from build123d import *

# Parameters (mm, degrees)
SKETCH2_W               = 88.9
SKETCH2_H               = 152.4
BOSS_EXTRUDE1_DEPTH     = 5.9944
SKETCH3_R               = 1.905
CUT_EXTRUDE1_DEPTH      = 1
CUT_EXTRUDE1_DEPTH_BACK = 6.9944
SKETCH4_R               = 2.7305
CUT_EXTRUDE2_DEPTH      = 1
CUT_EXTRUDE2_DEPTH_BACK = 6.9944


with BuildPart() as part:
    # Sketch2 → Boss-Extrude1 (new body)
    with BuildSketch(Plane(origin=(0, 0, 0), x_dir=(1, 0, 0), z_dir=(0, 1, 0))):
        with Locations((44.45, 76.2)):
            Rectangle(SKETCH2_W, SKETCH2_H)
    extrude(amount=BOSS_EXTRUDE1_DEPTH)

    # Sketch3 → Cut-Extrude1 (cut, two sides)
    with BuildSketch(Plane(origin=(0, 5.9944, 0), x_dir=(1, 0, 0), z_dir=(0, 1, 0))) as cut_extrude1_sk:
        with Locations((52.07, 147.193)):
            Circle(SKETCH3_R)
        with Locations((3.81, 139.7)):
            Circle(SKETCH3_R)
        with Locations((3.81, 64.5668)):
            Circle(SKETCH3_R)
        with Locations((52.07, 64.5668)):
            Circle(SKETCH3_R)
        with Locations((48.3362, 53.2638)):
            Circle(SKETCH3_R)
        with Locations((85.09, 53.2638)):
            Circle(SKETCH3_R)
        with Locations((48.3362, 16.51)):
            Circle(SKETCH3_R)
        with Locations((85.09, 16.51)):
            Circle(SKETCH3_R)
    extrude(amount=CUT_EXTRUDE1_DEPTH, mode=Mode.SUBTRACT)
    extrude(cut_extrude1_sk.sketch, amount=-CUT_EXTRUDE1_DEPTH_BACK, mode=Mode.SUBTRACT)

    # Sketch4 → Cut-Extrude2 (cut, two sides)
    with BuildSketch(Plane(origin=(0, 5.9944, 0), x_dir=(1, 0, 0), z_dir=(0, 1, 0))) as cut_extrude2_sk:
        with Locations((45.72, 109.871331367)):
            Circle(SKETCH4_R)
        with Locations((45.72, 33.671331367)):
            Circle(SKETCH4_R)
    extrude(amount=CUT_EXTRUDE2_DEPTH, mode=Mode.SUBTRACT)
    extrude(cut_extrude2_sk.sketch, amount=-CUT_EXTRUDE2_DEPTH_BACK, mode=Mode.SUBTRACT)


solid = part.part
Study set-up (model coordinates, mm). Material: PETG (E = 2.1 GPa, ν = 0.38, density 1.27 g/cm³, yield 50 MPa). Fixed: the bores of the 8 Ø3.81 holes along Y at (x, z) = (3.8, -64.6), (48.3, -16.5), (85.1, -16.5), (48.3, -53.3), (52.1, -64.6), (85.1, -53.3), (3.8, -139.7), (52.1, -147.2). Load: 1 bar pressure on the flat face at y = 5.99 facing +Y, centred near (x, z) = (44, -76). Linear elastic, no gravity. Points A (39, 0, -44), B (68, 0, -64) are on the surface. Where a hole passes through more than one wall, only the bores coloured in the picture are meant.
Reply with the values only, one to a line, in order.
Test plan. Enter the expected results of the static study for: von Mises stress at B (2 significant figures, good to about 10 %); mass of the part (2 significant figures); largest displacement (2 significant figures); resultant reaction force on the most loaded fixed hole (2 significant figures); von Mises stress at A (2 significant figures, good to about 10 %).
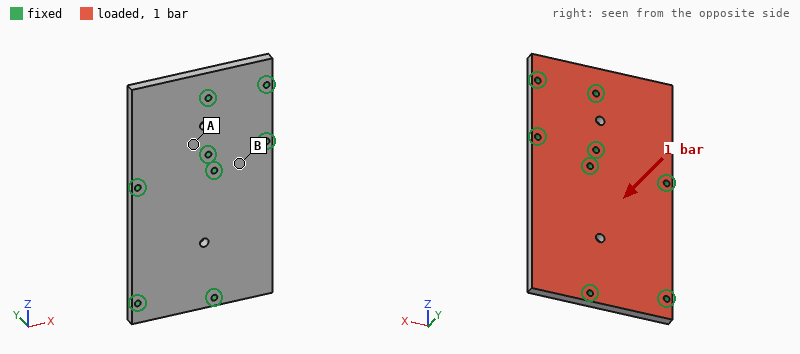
6.1 MPa
100 g
1.2 mm
290 N
2.4 MPa
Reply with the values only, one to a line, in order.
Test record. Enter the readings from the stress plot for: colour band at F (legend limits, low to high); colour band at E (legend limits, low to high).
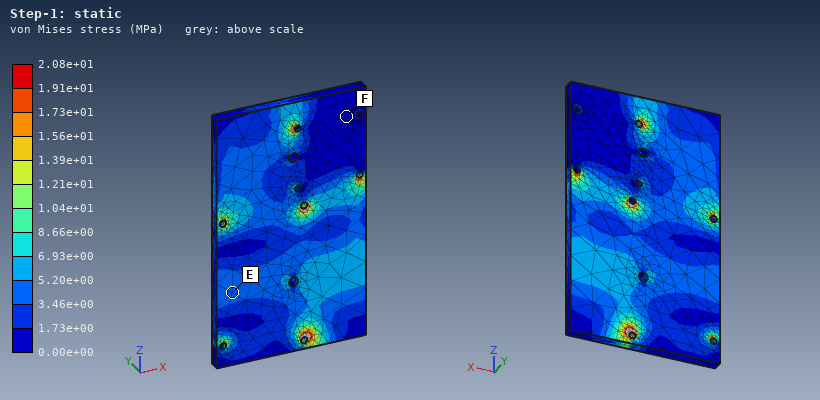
0.00e+00 to 1.73e+00 MPa
3.46e+00 to 5.20e+00 MPa
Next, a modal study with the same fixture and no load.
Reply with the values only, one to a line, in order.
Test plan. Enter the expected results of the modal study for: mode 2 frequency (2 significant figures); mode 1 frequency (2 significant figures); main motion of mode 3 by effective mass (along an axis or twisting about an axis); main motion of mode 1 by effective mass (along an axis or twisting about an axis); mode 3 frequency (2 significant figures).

760 Hz
710 Hz
along Y
along Y
1100 Hz
